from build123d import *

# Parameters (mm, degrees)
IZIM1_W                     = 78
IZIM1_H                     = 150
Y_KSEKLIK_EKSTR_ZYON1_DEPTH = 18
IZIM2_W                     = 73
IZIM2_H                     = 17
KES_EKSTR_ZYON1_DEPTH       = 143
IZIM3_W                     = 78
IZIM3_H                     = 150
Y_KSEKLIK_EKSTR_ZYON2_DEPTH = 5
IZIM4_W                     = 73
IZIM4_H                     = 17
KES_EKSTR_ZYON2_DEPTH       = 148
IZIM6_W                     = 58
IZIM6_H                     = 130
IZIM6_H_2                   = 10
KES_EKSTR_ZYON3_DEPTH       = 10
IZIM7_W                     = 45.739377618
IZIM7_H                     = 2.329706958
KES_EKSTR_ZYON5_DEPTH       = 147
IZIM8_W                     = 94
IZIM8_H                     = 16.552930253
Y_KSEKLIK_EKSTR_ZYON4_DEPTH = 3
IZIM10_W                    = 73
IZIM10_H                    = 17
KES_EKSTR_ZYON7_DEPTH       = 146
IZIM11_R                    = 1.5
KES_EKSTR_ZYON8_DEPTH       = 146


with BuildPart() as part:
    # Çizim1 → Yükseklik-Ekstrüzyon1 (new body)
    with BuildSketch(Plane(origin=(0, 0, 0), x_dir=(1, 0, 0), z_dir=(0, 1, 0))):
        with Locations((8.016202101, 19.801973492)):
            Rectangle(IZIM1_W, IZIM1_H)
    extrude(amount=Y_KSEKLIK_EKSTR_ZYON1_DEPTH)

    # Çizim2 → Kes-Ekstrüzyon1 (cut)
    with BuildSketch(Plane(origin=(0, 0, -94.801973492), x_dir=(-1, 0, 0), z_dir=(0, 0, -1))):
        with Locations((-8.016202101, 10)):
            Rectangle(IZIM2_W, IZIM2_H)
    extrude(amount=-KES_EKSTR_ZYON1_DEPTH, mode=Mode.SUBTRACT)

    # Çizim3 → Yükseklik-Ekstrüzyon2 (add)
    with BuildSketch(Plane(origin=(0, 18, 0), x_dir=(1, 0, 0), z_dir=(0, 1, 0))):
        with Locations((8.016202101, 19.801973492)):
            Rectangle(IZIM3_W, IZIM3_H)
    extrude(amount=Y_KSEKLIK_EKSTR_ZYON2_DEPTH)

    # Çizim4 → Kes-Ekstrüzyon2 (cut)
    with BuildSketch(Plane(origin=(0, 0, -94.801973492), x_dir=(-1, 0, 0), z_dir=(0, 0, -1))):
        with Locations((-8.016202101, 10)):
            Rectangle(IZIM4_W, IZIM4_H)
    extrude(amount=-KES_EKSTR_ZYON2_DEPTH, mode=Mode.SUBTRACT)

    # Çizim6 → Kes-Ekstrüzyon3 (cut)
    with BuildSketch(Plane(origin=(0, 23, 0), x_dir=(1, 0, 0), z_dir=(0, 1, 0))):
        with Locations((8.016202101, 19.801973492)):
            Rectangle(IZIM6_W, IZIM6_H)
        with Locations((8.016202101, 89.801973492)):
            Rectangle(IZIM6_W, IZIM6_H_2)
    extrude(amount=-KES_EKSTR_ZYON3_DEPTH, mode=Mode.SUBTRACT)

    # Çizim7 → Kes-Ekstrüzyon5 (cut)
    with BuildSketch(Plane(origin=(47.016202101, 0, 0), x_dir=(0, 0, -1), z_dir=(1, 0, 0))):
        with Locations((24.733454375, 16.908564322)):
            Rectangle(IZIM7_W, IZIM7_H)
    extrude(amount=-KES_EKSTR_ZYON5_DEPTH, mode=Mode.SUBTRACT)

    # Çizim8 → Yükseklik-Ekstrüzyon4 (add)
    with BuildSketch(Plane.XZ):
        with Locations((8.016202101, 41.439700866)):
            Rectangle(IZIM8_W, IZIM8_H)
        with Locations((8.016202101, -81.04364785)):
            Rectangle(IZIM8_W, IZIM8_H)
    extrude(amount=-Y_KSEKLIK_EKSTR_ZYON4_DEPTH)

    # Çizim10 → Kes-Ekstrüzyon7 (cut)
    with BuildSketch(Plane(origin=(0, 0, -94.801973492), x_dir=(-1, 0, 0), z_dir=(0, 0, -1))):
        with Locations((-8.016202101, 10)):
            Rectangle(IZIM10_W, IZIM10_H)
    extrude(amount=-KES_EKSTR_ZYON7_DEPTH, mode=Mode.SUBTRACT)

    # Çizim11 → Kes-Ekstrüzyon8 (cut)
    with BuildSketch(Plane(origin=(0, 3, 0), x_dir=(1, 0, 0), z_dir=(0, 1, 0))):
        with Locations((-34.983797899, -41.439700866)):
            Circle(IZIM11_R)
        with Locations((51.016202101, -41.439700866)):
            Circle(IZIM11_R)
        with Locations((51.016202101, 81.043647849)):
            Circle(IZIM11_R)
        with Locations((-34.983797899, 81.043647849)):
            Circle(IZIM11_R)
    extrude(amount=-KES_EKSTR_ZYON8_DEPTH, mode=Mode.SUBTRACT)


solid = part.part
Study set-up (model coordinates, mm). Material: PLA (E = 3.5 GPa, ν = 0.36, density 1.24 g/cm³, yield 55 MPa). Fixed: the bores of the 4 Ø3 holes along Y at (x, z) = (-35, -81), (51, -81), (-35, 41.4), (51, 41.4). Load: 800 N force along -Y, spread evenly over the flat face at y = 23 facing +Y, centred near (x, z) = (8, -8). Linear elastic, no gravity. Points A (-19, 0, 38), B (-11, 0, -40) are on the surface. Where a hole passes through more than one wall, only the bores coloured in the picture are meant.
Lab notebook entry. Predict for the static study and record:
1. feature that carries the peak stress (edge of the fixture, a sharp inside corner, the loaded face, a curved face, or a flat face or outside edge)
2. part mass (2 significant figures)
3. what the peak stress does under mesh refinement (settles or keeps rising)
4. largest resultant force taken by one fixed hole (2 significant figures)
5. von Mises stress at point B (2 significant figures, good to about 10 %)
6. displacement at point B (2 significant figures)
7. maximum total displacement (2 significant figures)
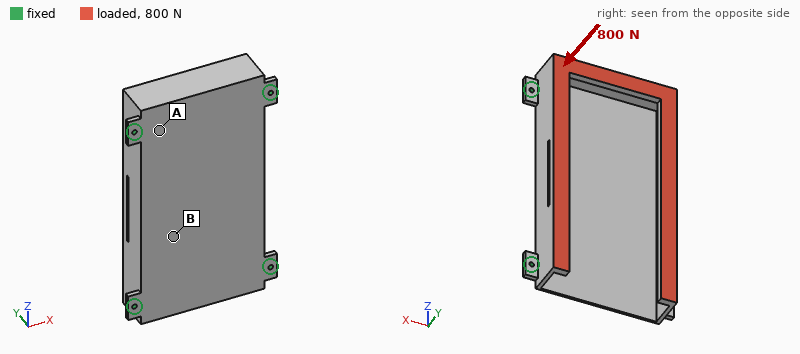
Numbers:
edge of the fixture
62 g
keeps rising
250 N
3.8 MPa
0.84 mm
1.5 mm
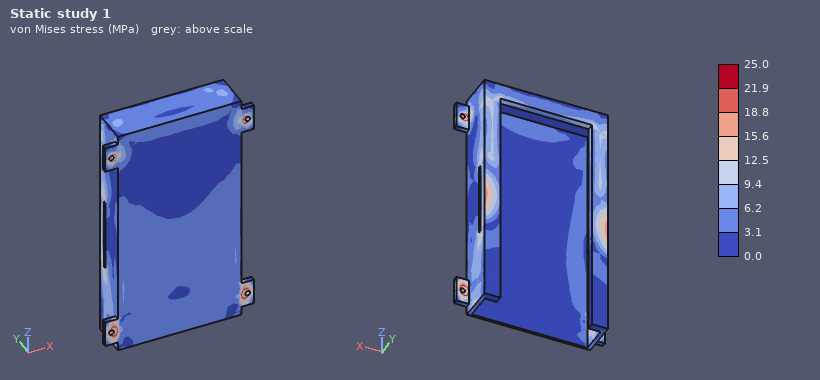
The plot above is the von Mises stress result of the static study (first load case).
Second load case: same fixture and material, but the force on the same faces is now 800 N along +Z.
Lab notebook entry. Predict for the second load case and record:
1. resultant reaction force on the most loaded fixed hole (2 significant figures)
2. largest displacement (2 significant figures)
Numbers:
220 N
0.37 mm
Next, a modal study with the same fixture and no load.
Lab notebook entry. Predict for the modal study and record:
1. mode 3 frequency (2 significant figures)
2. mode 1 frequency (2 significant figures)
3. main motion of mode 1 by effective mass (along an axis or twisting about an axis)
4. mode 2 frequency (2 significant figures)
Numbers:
530 Hz
360 Hz
along Y
520 Hz
